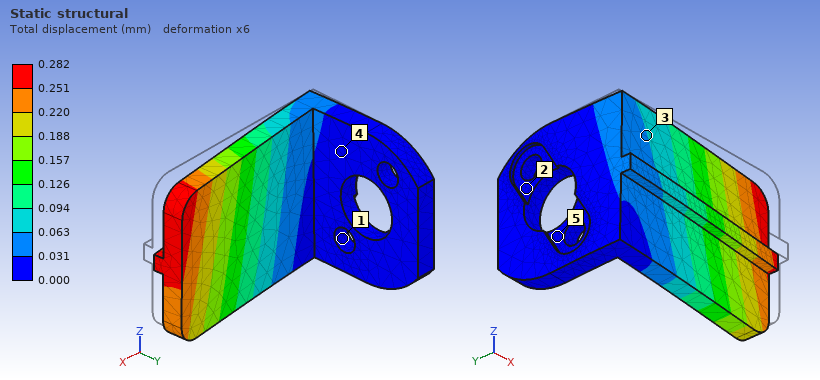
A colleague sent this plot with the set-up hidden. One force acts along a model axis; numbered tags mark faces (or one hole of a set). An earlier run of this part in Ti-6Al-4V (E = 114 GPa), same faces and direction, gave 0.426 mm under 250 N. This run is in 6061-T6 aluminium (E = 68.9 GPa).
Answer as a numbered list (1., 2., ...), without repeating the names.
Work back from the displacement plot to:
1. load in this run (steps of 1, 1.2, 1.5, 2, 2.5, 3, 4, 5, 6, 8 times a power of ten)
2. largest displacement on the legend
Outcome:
1. 100 N
2. 0.282 mm
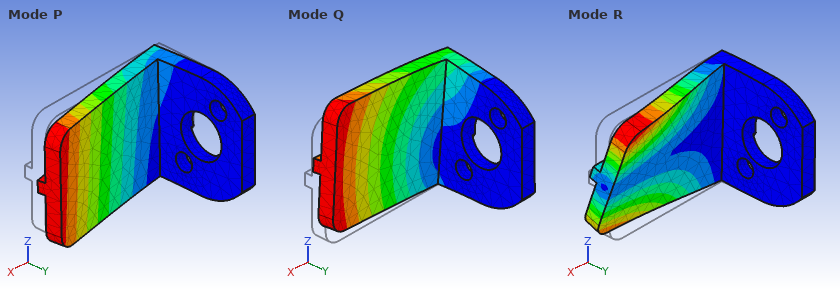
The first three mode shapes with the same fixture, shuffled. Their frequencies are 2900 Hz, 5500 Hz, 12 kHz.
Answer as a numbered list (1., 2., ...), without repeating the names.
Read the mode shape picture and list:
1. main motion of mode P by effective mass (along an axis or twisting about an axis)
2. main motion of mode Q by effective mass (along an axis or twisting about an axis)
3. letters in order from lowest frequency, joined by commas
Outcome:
1. along Y
2. along Z
3. P, Q, R
